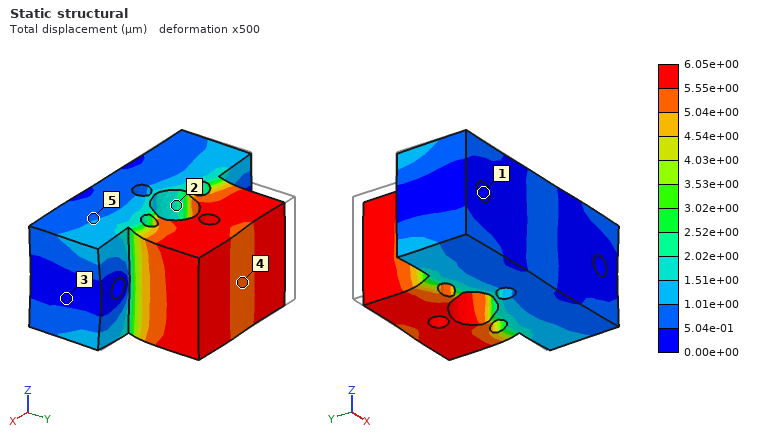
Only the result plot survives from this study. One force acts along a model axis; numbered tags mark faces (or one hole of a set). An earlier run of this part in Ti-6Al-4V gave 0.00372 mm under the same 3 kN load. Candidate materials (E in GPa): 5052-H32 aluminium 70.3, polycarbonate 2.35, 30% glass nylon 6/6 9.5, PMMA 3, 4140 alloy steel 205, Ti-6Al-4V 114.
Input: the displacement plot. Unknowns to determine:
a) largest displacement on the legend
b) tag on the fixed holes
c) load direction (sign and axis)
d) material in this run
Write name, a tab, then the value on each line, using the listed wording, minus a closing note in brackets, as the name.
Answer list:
largest displacement on the legend	6.05e+00 µm
tag on the fixed holes	1
load direction	+X
material in this run	5052-H32 aluminium
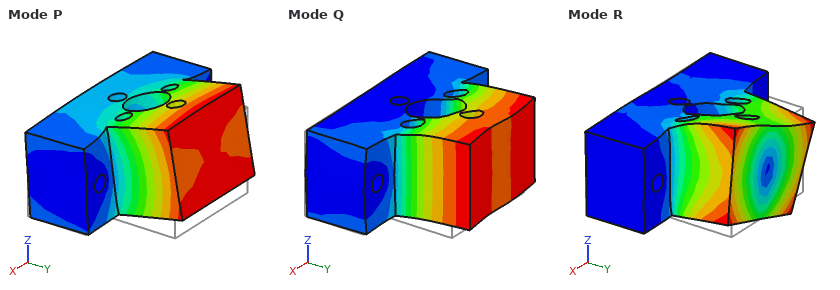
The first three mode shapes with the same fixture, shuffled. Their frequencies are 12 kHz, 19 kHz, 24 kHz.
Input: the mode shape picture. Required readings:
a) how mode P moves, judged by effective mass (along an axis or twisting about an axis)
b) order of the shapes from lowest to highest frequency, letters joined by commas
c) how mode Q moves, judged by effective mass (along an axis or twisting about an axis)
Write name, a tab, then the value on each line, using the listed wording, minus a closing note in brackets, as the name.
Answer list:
how mode P moves, judged by effective mass	along Z
order of the shapes from lowest to highest frequency, letters joined by commas	P, Q, R
how mode Q moves, judged by effective mass	along X
